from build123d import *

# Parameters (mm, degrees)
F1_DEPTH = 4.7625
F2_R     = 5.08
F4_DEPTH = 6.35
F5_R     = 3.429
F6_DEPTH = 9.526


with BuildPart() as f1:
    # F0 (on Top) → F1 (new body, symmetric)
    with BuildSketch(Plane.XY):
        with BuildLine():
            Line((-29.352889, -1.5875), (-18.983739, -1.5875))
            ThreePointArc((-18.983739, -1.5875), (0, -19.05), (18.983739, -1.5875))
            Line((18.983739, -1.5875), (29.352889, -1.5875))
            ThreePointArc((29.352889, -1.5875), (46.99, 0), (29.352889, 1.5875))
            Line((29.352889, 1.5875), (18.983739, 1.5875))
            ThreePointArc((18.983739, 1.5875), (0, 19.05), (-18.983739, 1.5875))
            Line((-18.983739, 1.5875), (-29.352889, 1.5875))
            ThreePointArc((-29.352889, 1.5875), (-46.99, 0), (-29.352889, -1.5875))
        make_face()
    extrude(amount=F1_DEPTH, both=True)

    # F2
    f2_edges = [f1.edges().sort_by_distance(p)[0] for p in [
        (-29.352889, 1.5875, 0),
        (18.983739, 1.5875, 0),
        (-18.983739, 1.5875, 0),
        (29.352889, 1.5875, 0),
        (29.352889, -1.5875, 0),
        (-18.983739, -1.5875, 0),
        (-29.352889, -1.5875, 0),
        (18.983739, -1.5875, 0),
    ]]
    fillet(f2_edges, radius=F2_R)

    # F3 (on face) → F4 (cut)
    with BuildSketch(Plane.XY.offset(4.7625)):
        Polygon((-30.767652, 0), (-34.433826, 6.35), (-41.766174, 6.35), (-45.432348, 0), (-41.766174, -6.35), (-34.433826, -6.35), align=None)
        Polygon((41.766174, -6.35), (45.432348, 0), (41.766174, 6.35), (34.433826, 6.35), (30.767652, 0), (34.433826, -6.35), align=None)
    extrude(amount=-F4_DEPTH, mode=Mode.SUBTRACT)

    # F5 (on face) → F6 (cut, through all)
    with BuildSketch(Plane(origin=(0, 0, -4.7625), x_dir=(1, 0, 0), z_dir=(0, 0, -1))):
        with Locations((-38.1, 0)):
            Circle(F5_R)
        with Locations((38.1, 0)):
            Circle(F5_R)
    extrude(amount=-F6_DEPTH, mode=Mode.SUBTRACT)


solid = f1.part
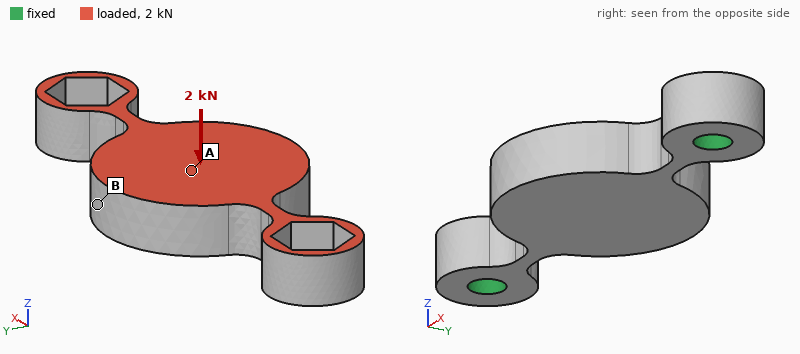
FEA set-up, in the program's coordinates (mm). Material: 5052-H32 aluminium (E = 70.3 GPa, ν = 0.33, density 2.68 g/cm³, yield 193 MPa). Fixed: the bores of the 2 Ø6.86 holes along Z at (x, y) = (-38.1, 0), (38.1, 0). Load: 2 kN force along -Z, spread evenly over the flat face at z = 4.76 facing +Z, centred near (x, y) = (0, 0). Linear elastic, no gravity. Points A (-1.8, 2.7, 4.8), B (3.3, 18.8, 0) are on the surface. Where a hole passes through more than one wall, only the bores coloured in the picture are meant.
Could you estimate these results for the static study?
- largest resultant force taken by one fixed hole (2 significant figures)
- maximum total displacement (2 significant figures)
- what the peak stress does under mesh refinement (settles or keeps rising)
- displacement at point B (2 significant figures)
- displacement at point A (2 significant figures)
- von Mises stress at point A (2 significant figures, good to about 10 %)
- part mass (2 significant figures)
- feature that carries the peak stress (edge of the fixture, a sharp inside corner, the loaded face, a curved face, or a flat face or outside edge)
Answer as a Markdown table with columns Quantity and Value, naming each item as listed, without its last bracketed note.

| Quantity | Value |
|---|---|
| largest resultant force taken by one fixed hole | 1.4 kN |
| maximum total displacement | 90 µm |
| what the peak stress does under mesh refinement | keeps rising |
| displacement at point B | 90 µm |
| displacement at point A | 83 µm |
| von Mises stress at point A | 38 MPa |
| part mass | 39 g |
| feature that carries the peak stress | edge of the fixture |
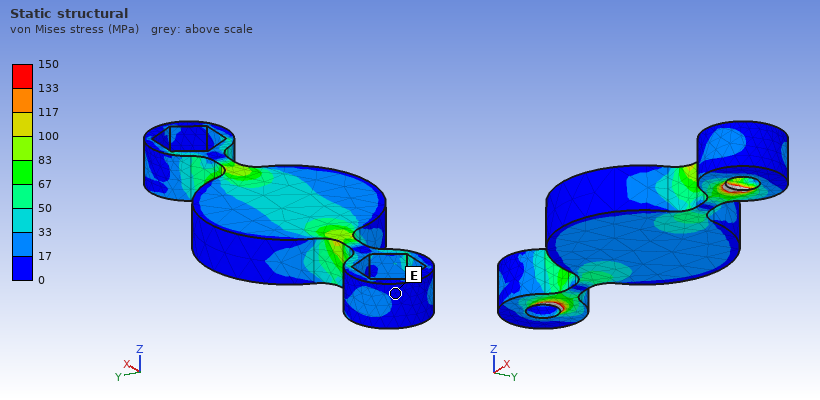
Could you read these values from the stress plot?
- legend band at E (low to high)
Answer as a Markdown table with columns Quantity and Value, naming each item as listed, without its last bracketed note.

| Quantity | Value |
|---|---|
| legend band at E | 0 to 17 MPa |
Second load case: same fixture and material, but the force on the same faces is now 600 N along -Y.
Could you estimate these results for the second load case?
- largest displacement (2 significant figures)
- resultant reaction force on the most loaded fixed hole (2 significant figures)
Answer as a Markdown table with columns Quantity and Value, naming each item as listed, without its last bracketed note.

| Quantity | Value |
|---|---|
| largest displacement | 79 µm |
| resultant reaction force on the most loaded fixed hole | 300 N |
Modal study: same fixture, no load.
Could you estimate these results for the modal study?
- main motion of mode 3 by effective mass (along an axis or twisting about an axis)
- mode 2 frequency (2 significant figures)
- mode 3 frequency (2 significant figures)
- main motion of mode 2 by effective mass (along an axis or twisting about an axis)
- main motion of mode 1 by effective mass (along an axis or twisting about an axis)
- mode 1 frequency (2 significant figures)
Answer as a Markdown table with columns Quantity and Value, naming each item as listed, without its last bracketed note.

| Quantity | Value |
|---|---|
| main motion of mode 3 by effective mass | along Y |
| mode 2 frequency | 4100 Hz |
| mode 3 frequency | 5000 Hz |
| main motion of mode 2 by effective mass | along Z |
| main motion of mode 1 by effective mass | twisting about X |
| mode 1 frequency | 2500 Hz |
